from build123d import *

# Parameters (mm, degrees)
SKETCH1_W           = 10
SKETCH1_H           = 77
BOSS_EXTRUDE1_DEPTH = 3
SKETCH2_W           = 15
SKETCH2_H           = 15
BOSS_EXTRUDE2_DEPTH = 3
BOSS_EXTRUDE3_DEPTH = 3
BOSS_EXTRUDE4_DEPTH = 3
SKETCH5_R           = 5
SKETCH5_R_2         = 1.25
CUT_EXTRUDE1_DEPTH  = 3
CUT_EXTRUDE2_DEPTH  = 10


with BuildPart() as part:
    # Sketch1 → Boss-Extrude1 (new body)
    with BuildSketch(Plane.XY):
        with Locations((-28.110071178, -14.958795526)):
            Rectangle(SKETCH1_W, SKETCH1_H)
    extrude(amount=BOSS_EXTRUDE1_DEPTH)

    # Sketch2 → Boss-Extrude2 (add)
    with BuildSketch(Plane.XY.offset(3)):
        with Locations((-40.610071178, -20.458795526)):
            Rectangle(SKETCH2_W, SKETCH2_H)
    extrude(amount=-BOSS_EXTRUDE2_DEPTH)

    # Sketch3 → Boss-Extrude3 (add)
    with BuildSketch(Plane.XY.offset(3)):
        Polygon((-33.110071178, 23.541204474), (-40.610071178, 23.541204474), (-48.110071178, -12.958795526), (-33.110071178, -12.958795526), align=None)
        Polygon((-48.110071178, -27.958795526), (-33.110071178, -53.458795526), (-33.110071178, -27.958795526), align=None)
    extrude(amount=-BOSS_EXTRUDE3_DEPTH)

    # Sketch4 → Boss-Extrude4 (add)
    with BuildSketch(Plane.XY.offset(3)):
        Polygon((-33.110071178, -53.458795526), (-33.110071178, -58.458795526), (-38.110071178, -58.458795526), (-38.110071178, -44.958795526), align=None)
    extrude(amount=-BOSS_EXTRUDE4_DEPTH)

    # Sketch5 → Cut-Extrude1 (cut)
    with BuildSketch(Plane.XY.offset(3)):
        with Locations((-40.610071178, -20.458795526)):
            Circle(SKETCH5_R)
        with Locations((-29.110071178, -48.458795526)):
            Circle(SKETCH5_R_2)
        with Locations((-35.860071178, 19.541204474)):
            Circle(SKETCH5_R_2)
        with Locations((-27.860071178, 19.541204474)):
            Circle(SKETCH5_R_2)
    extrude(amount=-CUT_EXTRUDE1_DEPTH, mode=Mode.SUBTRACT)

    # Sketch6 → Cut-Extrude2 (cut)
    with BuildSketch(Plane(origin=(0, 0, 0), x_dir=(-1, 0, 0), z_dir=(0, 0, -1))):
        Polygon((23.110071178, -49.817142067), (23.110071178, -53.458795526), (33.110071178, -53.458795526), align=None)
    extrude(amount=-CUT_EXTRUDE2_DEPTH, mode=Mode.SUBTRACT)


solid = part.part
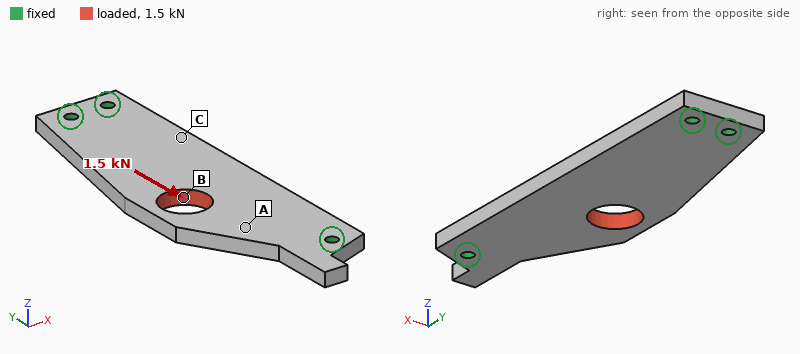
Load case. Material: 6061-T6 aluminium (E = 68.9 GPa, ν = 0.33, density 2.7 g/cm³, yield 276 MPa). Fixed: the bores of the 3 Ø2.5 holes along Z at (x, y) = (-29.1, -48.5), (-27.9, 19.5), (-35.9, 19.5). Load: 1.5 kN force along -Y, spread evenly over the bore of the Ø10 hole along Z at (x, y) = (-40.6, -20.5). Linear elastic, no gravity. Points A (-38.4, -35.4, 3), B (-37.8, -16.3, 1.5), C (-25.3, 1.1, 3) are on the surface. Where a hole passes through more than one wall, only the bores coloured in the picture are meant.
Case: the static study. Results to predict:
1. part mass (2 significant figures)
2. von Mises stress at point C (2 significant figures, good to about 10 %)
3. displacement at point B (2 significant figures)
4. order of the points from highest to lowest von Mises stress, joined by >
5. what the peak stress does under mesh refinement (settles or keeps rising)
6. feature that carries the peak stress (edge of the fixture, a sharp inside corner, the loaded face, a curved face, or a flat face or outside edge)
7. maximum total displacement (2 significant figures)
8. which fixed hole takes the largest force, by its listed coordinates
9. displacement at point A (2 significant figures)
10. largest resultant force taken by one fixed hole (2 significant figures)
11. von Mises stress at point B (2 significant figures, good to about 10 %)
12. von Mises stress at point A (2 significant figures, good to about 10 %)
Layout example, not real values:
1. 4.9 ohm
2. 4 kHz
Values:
1. 12 g
2. 7.1 MPa
3. 7.8 µm
4. B > A > C
5. keeps rising
6. edge of the fixture
7. 13 µm
8. (-29.1, -48.5)
9. 7.0 µm
10. 730 N
11. 27 MPa
12. 15 MPa
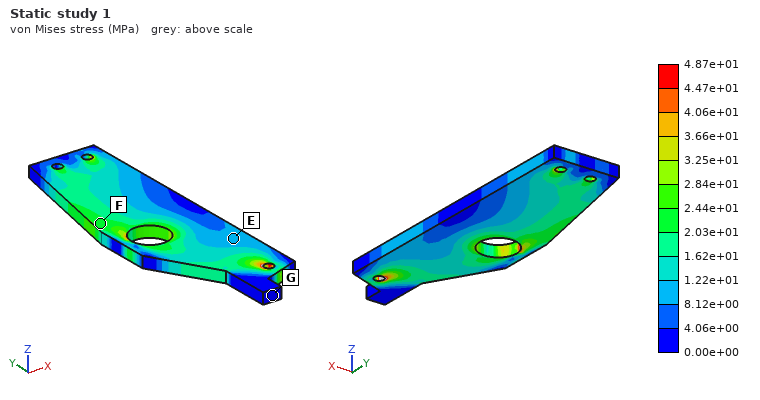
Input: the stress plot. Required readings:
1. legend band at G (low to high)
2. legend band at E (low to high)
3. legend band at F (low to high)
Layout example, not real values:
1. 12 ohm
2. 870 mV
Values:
1. 0.00e+00 to 4.06e+00 MPa
2. 8.12e+00 to 1.22e+01 MPa
3. 2.03e+01 to 2.44e+01 MPa
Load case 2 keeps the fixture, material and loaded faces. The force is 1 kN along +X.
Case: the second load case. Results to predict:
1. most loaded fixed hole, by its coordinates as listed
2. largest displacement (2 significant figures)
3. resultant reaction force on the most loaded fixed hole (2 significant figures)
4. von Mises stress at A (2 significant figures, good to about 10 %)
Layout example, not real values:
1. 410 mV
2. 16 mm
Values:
1. (-27.9, 19.5)
2. 30 µm
3. 770 N
4. 21 MPa
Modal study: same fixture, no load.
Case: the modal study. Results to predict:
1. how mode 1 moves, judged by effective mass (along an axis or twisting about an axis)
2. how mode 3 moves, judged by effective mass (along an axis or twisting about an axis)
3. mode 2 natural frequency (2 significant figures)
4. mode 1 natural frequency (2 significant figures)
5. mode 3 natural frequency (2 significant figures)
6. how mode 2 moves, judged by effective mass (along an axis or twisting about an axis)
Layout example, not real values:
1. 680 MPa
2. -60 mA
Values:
1. along Z
2. twisting about X
3. 5400 Hz
4. 2900 Hz
5. 8100 Hz
6. twisting about Y
